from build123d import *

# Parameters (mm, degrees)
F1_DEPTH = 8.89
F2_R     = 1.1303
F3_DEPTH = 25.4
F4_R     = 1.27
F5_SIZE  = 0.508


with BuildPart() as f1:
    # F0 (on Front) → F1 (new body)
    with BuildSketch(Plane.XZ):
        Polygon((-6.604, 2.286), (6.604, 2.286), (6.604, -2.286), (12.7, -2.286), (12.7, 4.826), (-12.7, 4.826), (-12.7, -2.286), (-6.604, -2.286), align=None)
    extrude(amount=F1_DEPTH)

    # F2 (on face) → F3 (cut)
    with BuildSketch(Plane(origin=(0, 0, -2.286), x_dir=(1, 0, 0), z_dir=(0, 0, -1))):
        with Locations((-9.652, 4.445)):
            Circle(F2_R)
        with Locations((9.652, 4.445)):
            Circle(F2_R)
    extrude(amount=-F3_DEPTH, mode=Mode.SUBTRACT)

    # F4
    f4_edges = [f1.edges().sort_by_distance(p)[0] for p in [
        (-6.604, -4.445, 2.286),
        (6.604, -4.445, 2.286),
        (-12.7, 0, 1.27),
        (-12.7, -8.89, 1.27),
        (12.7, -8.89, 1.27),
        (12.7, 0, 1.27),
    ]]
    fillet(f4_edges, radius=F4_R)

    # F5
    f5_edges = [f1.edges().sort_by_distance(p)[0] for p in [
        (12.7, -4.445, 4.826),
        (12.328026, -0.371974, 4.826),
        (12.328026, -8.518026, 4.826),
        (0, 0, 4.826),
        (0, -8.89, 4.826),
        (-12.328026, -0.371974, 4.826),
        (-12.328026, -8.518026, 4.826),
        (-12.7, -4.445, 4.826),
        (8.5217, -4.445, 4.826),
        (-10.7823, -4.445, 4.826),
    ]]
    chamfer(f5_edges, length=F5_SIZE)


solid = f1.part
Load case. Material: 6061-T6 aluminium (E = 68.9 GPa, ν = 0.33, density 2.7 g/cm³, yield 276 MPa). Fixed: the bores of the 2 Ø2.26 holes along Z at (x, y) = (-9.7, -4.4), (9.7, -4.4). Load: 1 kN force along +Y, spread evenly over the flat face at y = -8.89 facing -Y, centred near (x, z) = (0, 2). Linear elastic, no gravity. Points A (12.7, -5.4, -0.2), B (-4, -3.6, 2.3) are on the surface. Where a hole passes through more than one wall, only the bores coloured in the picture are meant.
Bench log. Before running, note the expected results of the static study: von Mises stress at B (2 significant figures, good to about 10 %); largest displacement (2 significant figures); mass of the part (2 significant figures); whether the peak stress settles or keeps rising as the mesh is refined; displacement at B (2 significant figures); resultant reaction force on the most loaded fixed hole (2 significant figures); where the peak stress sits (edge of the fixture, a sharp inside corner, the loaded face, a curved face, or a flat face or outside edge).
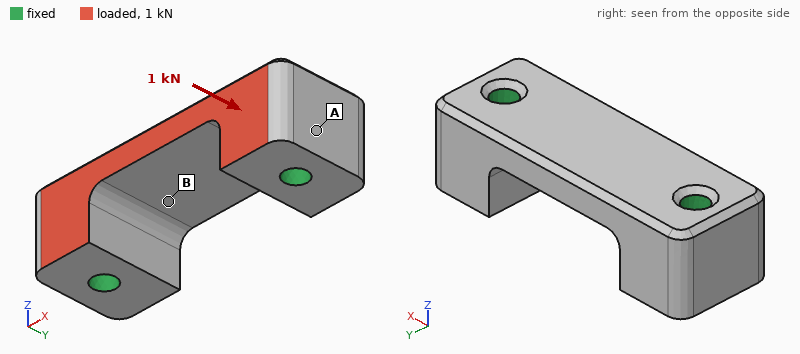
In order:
12 MPa
3.6 µm
2.7 g
keeps rising
2.4 µm
500 N
edge of the fixture
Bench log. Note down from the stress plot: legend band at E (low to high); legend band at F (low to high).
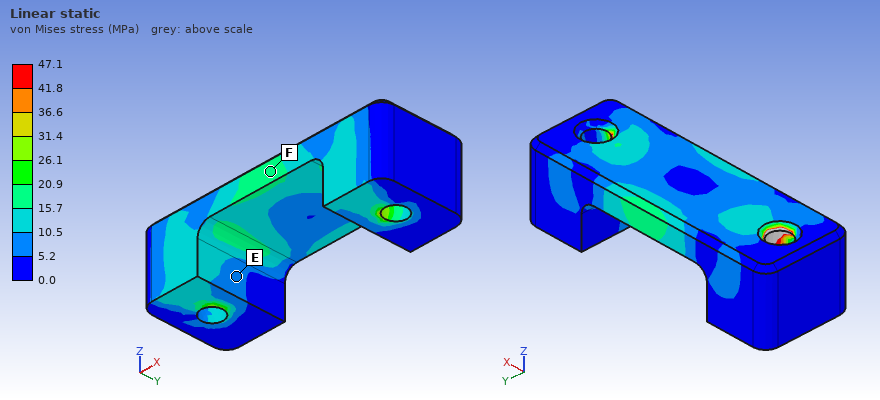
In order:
5.2 to 10.5 MPa
15.7 to 20.9 MPa
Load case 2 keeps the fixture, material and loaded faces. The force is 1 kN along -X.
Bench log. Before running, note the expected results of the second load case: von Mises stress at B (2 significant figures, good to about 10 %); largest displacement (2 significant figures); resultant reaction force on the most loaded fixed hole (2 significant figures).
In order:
12 MPa
4.1 µm
520 N
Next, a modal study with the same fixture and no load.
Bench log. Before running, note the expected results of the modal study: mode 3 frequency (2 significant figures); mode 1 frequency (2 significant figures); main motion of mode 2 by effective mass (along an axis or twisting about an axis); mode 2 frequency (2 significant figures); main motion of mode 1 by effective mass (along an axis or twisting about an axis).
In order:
66 kHz
49 kHz
along Y
59 kHz
along Z
